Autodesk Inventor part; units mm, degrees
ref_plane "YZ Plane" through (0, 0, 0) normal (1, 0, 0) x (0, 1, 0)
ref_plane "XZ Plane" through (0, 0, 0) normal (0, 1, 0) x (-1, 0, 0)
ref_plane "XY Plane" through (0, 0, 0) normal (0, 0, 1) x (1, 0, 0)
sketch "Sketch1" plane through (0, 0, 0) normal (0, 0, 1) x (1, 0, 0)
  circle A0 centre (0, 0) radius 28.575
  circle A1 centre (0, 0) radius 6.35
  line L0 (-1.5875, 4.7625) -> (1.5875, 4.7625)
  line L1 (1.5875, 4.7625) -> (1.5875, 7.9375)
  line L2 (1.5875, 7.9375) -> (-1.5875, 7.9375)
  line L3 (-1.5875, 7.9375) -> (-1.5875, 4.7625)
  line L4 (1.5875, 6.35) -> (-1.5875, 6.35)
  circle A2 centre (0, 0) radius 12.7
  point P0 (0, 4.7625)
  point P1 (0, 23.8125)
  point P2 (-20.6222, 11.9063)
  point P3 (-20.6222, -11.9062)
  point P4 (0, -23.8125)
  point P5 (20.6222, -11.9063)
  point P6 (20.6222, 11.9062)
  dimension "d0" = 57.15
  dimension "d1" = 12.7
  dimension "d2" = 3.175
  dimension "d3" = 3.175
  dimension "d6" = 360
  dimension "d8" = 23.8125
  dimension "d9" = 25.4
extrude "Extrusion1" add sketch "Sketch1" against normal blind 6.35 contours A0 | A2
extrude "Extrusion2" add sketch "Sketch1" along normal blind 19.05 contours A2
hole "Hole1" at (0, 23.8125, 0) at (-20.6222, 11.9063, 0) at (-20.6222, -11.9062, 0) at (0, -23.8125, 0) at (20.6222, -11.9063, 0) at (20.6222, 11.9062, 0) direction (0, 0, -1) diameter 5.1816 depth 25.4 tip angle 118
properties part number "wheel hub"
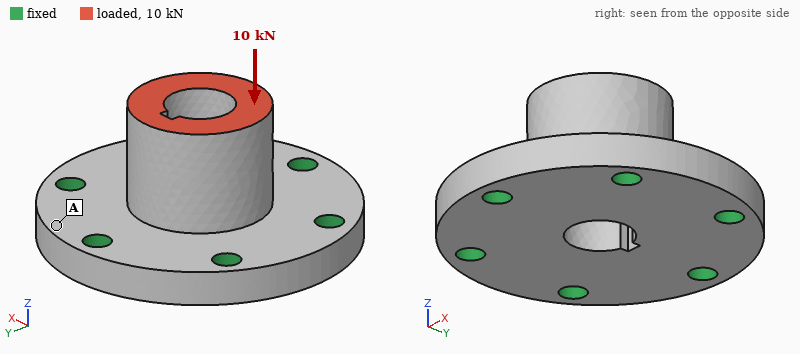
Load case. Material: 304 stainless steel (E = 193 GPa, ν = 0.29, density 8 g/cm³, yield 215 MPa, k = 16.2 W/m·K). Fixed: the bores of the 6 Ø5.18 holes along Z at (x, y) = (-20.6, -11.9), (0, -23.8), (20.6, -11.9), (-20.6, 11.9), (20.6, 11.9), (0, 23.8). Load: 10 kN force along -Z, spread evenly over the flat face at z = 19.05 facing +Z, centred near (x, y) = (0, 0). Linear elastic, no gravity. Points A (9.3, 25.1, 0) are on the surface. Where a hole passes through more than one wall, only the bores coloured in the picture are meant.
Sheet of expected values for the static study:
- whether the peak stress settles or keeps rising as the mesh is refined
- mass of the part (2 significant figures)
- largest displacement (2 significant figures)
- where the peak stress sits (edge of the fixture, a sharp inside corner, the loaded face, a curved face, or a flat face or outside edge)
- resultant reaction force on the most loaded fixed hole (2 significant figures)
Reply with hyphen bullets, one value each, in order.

- keeps rising
- 170 g
- 12 µm
- edge of the fixture
- 1.8 kN
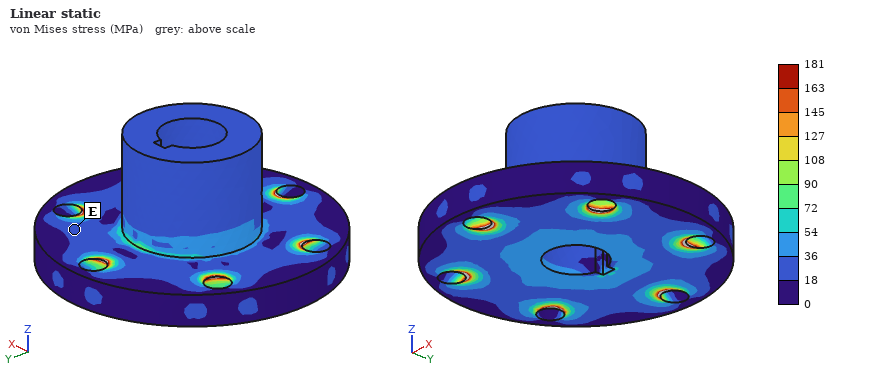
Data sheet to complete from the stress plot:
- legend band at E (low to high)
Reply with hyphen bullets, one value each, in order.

- 18 to 36 MPa
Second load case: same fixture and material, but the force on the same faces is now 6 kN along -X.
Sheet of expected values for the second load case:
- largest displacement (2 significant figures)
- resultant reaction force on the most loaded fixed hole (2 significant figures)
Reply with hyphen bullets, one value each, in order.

- 31 µm
- 2.5 kN
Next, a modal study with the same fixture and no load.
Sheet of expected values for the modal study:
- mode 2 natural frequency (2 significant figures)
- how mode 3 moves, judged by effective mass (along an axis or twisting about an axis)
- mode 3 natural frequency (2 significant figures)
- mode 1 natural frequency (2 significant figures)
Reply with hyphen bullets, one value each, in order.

- 15 kHz
- along Z
- 17 kHz
- 15 kHz
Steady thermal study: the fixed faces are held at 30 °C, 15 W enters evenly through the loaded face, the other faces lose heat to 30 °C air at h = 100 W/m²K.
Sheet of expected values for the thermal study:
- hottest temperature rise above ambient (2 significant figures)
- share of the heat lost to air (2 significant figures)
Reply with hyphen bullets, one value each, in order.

- 47 K
- 54 %
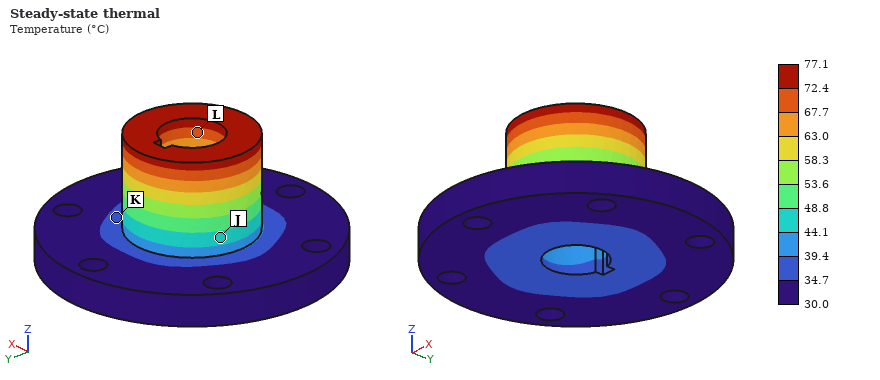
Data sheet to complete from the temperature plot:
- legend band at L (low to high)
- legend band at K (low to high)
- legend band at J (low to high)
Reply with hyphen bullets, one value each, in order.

- 67.7 to 72.4 °C
- 34.7 to 39.4 °C
- 44.1 to 48.8 °C
